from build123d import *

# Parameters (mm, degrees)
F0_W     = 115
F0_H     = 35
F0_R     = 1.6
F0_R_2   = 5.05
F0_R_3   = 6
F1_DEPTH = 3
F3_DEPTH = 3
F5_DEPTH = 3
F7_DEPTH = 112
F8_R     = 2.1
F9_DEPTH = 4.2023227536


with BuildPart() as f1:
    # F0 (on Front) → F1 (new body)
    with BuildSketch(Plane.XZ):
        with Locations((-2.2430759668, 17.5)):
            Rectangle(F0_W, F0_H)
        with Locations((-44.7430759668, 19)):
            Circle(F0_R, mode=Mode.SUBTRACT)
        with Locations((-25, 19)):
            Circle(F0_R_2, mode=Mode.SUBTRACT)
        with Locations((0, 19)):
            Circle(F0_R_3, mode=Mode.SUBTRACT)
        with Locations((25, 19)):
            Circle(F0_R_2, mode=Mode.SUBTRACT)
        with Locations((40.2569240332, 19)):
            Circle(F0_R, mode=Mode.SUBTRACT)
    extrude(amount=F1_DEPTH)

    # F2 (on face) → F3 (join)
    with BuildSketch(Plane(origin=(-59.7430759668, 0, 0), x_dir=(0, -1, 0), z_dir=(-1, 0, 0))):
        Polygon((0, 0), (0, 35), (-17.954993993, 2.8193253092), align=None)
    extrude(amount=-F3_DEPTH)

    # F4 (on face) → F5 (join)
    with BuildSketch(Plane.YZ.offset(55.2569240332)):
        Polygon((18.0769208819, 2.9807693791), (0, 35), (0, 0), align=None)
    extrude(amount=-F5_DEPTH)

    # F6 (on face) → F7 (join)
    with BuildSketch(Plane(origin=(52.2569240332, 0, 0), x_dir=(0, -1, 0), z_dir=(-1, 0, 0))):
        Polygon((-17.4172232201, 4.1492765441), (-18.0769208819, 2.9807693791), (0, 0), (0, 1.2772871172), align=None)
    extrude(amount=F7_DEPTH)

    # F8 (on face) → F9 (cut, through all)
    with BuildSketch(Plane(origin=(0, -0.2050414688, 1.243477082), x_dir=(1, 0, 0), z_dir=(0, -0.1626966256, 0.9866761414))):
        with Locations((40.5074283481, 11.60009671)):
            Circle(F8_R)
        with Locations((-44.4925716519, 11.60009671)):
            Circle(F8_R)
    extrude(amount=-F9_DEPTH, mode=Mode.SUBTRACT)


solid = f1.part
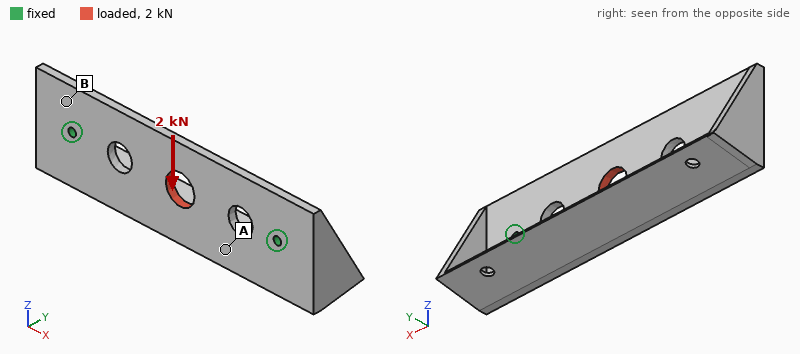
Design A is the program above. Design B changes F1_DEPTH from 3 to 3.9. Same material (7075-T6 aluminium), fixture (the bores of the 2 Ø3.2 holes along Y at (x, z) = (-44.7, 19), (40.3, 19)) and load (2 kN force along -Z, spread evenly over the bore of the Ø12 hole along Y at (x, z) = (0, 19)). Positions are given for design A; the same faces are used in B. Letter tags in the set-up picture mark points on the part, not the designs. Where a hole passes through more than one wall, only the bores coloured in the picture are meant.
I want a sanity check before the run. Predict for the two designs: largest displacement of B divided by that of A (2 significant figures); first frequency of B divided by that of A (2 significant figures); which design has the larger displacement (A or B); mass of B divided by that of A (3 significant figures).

0.77
1.2
A
1.22
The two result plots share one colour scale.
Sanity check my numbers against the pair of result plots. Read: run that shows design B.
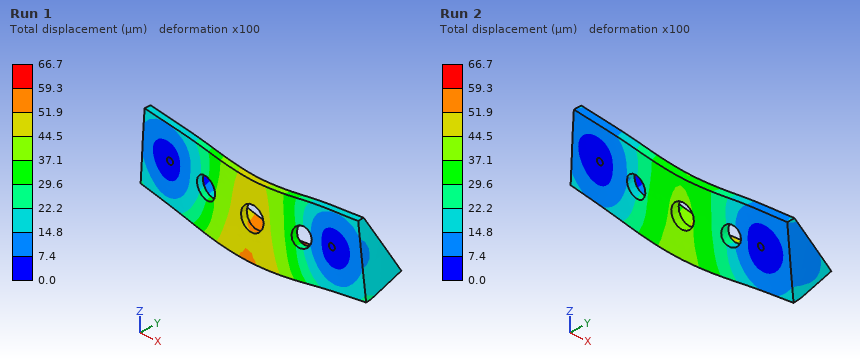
Run 2
